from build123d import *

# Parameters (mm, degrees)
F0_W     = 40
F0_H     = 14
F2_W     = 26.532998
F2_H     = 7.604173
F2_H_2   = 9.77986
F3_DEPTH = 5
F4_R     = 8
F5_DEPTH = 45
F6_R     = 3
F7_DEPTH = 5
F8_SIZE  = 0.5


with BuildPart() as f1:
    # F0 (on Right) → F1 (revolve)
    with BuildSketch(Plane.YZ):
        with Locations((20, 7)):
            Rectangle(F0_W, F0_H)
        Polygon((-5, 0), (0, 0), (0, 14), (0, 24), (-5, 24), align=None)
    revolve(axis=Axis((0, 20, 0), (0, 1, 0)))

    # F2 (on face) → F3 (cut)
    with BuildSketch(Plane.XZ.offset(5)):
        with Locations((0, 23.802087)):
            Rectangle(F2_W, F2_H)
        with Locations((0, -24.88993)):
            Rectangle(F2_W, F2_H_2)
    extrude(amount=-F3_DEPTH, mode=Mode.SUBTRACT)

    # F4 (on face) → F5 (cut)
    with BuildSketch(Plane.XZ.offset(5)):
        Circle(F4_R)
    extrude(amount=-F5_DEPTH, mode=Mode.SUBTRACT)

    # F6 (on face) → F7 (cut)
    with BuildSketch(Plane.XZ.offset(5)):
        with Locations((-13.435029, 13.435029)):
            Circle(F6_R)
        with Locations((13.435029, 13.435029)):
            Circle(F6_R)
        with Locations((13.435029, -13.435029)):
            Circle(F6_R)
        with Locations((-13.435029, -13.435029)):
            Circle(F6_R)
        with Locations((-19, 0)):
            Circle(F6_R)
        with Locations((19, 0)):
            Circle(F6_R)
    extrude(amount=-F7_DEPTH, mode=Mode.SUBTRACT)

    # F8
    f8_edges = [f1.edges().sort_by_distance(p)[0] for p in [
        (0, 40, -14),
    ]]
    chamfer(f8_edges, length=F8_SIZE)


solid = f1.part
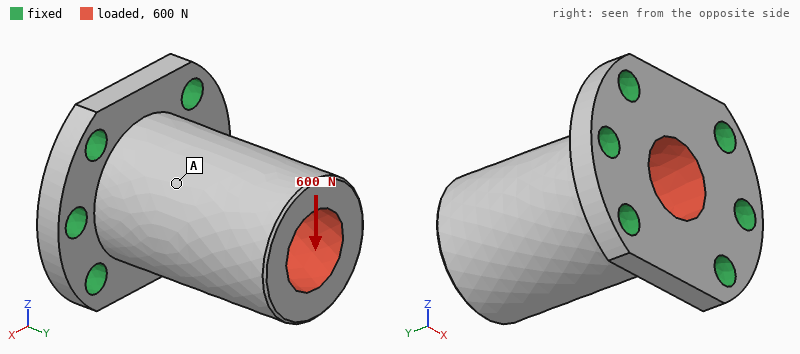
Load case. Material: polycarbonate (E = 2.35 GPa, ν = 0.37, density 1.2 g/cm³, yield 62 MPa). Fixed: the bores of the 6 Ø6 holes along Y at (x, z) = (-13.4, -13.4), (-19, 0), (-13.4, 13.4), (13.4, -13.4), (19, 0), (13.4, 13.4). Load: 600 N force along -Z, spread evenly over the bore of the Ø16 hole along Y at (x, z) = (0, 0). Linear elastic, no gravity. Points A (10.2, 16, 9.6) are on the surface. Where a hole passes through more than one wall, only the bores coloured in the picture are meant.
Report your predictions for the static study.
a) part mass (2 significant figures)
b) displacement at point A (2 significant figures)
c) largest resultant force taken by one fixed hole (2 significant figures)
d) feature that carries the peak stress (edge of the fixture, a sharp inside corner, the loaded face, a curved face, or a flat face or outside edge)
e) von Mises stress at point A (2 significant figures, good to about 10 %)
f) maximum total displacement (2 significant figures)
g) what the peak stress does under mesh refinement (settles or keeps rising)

28 g
0.11 mm
290 N
edge of the fixture
1.9 MPa
0.26 mm
keeps rising
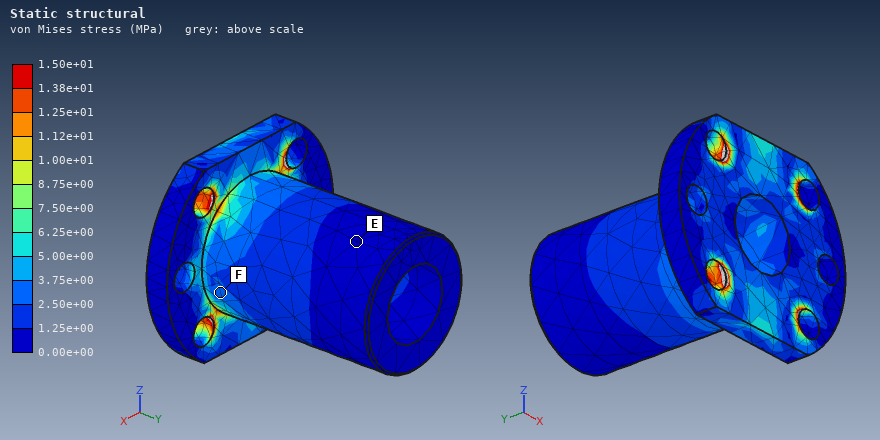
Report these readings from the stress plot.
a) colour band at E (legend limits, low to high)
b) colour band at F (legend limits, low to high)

0.00e+00 to 1.25e+00 MPa
2.50e+00 to 3.75e+00 MPa
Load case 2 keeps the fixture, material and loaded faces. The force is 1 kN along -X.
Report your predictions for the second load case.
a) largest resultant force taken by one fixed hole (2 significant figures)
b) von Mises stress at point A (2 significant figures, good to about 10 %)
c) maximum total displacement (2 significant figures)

390 N
3.2 MPa
0.32 mm
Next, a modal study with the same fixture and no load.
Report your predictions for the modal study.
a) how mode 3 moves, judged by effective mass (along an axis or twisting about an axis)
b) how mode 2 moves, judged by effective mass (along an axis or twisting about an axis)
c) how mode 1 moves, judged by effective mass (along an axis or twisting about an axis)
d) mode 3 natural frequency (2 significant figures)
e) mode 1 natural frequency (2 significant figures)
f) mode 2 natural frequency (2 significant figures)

twisting about Y
along X
along Z
4800 Hz
1900 Hz
2200 Hz
